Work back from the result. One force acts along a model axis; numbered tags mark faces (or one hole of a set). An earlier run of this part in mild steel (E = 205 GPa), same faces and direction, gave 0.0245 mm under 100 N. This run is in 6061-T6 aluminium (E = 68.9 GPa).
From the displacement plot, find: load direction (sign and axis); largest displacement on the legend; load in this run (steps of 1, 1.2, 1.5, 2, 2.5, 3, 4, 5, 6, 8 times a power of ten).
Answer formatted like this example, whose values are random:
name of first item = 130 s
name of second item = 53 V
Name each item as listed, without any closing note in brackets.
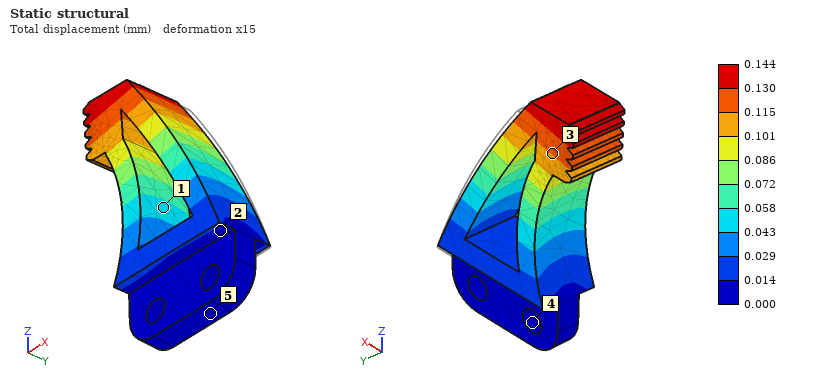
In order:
load direction = -Y
largest displacement on the legend = 0.144 mm
load in this run = 200 N
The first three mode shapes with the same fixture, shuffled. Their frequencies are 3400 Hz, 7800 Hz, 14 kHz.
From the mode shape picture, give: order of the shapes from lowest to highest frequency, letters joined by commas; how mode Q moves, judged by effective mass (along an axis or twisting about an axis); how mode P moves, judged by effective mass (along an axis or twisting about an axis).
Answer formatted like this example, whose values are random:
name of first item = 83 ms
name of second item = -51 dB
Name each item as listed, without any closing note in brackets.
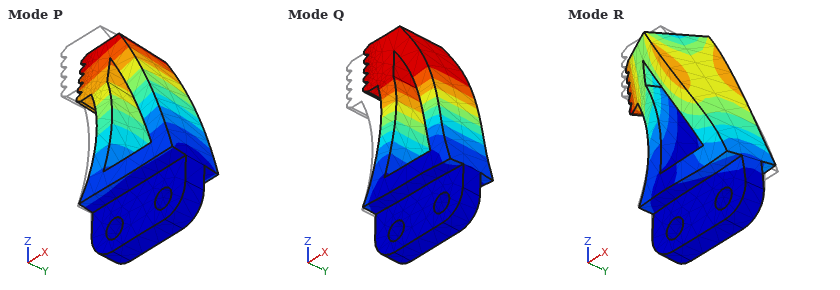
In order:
order of the shapes from lowest to highest frequency, letters joined by commas = P, Q, R
how mode Q moves, judged by effective mass = along X
how mode P moves, judged by effective mass = along Y
